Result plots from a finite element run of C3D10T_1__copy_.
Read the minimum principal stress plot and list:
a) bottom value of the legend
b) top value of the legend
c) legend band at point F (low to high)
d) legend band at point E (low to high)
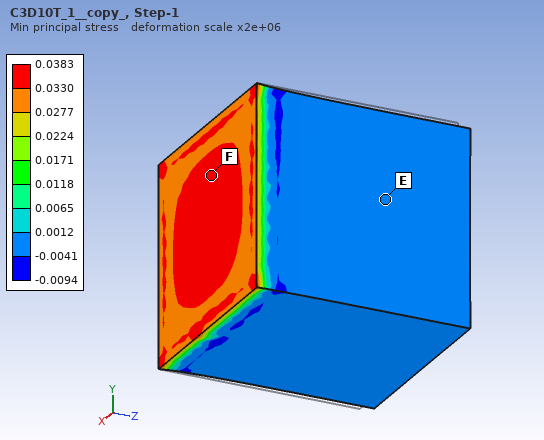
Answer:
-0.0094
0.0383
0.0330 to 0.0383
-0.0041 to 0.0012
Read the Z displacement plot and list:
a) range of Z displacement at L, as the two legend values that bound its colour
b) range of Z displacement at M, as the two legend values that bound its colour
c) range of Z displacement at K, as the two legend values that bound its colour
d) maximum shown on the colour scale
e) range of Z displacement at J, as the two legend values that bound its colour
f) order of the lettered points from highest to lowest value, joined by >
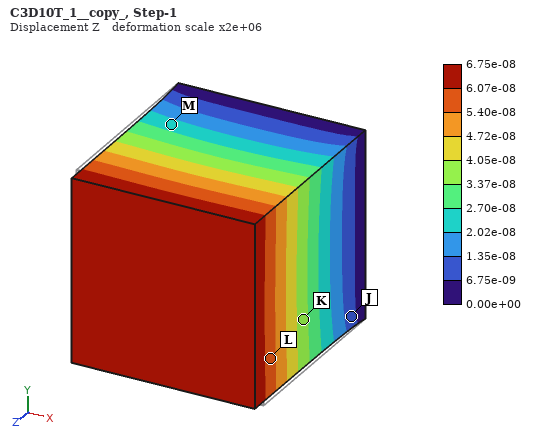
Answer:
5.40e-08 to 6.07e-08
2.02e-08 to 2.70e-08
3.37e-08 to 4.05e-08
6.75e-08
6.75e-09 to 1.35e-08
L > K > M > J
